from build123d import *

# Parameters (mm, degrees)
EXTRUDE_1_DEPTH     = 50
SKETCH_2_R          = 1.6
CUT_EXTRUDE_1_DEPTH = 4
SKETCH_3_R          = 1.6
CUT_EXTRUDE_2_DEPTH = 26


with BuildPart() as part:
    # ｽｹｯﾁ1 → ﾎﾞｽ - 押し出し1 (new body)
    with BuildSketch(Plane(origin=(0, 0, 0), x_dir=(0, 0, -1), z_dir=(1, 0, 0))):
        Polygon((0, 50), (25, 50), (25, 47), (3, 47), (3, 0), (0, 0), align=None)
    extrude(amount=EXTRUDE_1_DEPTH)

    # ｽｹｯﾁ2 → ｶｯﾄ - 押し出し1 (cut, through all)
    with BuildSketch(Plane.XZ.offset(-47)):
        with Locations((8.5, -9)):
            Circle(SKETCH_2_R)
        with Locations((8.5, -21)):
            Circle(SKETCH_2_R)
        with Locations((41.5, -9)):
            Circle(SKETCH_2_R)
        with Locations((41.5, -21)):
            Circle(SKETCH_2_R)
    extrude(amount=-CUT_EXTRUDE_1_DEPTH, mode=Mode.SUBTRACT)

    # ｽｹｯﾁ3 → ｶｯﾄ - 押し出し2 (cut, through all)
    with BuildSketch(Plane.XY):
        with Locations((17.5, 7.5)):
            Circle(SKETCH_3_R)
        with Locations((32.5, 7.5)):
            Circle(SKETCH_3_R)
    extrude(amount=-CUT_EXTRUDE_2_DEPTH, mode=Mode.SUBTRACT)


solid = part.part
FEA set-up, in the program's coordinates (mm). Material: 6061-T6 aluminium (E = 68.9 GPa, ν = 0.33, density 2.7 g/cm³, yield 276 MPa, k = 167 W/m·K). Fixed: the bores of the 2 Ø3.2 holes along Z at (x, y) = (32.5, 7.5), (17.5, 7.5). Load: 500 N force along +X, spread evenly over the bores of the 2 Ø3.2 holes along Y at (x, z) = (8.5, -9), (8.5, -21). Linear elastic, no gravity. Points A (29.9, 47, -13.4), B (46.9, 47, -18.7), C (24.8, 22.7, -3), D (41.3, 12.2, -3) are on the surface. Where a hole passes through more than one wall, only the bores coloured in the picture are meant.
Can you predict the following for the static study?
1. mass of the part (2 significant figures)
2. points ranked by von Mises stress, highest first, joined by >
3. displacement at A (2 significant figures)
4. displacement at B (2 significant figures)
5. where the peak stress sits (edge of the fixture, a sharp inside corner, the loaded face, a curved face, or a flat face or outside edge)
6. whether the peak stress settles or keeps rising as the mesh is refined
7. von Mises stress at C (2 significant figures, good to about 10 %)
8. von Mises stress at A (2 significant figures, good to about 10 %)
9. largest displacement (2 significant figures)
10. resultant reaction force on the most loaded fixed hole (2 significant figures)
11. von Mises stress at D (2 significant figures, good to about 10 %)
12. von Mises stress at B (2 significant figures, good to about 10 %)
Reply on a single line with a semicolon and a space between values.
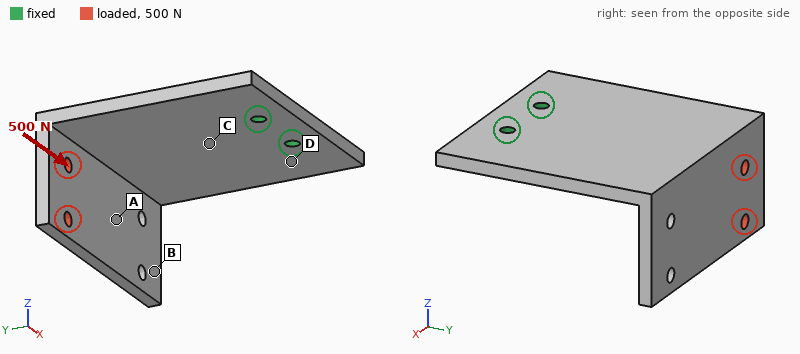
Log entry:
29 g; C > D > A > B; 0.27 mm; 0.52 mm; edge of the fixture; keeps rising; 89 MPa; 24 MPa; 0.65 mm; 1.2 kN; 43 MPa; 12 MPa
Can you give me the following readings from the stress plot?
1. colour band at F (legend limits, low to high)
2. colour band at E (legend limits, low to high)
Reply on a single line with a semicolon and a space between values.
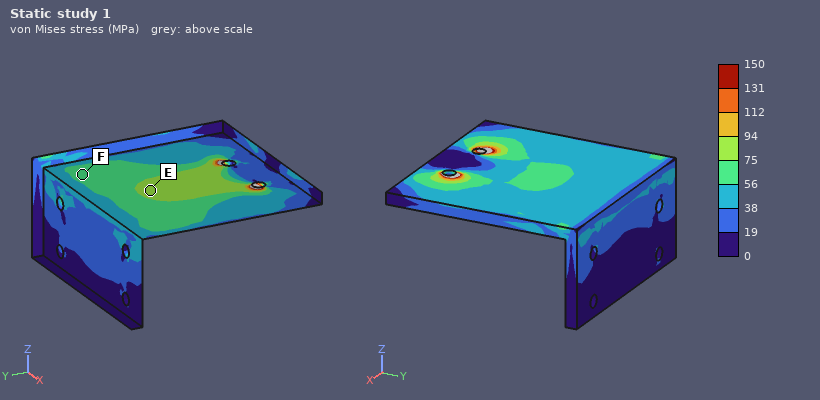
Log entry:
56 to 75 MPa; 75 to 94 MPa
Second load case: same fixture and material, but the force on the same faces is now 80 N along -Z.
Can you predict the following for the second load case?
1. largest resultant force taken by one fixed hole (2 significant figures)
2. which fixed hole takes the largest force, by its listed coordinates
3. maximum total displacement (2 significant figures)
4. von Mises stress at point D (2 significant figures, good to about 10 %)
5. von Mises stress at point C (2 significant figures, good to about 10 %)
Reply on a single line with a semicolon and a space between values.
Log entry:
95 N; (17.5, 7.5); 0.43 mm; 23 MPa; 30 MPa
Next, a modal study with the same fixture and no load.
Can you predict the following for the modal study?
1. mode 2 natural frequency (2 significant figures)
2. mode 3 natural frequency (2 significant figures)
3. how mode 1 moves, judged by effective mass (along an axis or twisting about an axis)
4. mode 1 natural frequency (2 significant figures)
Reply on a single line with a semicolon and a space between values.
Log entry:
1400 Hz; 2700 Hz; along Z; 710 Hz
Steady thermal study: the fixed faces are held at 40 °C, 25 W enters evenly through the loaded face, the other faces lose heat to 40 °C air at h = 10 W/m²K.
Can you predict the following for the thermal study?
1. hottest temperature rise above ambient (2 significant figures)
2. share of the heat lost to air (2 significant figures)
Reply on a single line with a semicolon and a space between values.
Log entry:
75 K; 9.4 %
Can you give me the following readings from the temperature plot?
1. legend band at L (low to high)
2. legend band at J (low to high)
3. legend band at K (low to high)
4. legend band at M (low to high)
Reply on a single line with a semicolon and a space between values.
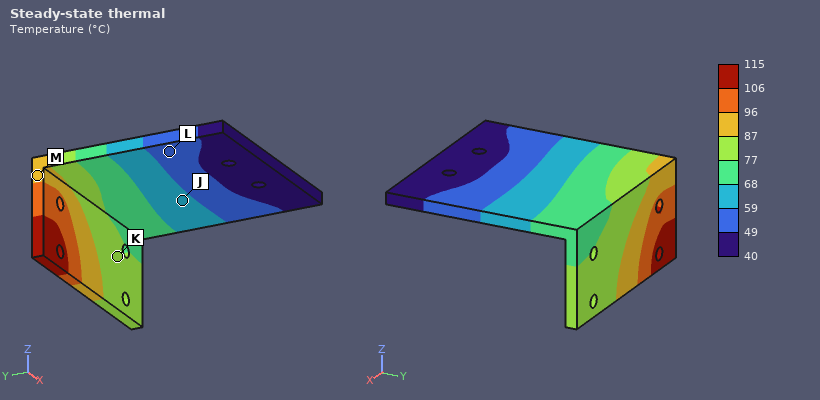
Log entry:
49 to 59 °C; 59 to 68 °C; 77 to 87 °C; 87 to 96 °C
